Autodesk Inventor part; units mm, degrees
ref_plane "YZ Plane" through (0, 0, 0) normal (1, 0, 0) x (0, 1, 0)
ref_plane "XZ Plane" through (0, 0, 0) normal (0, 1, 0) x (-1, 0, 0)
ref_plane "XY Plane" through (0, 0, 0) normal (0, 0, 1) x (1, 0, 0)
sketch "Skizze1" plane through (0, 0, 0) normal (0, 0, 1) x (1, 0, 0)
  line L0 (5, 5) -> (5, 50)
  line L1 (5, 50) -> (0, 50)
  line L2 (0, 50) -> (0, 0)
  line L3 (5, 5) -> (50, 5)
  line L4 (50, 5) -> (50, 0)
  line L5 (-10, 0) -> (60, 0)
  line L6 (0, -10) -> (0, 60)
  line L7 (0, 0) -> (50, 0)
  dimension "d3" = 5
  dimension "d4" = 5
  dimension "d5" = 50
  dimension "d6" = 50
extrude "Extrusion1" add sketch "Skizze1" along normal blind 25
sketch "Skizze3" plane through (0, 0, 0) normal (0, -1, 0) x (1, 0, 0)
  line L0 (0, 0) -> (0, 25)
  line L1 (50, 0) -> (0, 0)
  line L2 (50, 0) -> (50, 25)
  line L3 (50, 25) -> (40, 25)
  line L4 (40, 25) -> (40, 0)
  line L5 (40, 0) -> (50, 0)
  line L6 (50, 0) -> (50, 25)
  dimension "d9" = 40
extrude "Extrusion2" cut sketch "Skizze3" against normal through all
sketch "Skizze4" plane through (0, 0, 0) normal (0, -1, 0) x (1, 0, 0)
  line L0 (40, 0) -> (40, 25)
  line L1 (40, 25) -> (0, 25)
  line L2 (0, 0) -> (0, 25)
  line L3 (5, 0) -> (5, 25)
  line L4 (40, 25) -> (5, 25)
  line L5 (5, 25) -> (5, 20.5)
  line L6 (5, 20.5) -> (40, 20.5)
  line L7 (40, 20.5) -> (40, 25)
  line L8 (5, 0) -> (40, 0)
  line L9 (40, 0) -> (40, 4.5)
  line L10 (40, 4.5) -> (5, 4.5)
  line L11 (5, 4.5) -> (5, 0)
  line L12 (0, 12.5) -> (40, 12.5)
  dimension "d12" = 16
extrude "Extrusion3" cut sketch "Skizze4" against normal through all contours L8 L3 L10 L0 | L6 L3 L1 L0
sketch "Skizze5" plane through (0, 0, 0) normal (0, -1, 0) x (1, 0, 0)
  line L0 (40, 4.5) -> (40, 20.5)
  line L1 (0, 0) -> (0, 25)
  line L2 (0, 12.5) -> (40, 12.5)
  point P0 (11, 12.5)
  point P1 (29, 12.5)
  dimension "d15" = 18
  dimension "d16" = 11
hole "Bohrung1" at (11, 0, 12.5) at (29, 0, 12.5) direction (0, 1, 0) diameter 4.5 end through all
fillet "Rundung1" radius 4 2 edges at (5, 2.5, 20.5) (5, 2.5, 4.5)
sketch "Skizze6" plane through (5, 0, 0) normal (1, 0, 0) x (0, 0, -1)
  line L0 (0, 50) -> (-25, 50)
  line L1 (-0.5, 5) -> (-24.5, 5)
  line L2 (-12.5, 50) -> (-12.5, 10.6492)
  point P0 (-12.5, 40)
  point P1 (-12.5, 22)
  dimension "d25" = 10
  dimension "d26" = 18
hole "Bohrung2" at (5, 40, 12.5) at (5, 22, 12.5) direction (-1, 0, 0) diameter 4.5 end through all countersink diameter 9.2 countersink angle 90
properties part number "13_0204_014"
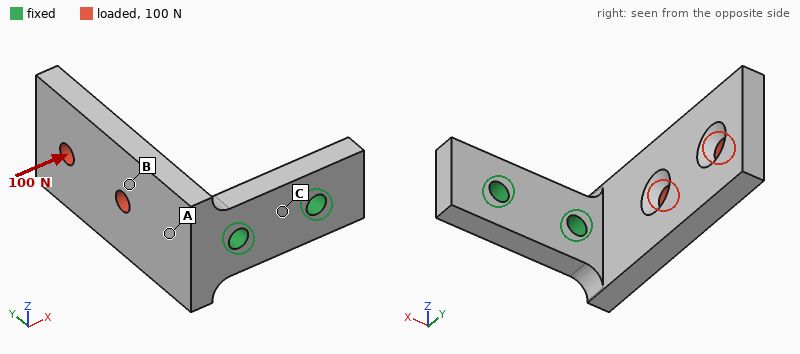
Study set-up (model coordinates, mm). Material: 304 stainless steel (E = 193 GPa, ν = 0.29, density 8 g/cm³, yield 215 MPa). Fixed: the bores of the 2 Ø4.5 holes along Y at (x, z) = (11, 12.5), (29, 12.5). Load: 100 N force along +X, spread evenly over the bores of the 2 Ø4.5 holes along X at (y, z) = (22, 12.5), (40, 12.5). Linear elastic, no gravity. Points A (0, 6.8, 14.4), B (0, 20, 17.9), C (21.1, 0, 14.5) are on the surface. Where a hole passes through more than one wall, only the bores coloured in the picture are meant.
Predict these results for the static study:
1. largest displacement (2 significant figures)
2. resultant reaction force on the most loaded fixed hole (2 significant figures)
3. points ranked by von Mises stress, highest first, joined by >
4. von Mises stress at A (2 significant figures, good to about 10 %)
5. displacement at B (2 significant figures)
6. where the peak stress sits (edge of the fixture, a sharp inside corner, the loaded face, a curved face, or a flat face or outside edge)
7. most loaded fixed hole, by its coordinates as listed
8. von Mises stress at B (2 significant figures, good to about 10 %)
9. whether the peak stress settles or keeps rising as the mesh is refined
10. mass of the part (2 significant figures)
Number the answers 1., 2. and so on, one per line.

1. 60 µm
2. 98 N
3. A > B > C
4. 24 MPa
5. 17 µm
6. edge of the fixture
7. (11, 12.5)
8. 13 MPa
9. keeps rising
10. 69 g
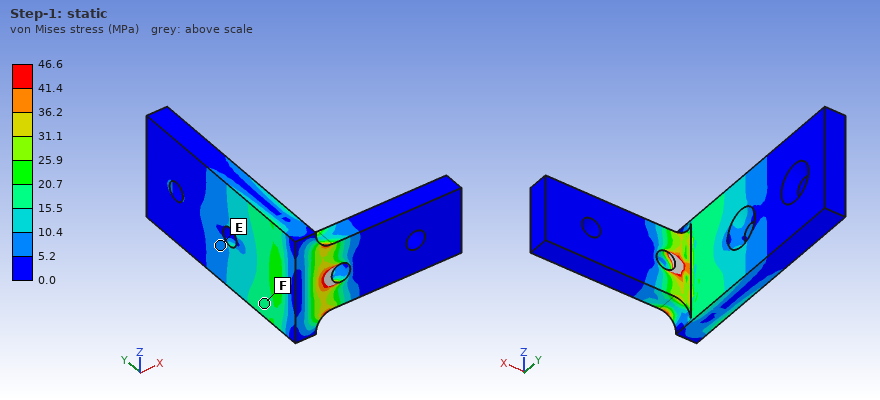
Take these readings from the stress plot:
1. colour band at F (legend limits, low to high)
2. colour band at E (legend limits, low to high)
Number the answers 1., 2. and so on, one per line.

1. 15.5 to 20.7 MPa
2. 5.2 to 10.4 MPa
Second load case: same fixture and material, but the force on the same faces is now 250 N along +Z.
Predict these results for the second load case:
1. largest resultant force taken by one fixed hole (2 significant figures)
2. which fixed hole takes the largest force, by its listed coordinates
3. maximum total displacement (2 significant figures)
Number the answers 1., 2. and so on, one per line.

1. 320 N
2. (11, 12.5)
3. 49 µm
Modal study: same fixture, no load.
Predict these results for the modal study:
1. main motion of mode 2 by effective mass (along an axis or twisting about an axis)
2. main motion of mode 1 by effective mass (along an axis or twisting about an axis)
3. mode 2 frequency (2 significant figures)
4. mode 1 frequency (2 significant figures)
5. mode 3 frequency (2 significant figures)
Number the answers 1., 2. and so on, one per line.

1. along Z
2. along X
3. 2200 Hz
4. 1300 Hz
5. 5800 Hz
